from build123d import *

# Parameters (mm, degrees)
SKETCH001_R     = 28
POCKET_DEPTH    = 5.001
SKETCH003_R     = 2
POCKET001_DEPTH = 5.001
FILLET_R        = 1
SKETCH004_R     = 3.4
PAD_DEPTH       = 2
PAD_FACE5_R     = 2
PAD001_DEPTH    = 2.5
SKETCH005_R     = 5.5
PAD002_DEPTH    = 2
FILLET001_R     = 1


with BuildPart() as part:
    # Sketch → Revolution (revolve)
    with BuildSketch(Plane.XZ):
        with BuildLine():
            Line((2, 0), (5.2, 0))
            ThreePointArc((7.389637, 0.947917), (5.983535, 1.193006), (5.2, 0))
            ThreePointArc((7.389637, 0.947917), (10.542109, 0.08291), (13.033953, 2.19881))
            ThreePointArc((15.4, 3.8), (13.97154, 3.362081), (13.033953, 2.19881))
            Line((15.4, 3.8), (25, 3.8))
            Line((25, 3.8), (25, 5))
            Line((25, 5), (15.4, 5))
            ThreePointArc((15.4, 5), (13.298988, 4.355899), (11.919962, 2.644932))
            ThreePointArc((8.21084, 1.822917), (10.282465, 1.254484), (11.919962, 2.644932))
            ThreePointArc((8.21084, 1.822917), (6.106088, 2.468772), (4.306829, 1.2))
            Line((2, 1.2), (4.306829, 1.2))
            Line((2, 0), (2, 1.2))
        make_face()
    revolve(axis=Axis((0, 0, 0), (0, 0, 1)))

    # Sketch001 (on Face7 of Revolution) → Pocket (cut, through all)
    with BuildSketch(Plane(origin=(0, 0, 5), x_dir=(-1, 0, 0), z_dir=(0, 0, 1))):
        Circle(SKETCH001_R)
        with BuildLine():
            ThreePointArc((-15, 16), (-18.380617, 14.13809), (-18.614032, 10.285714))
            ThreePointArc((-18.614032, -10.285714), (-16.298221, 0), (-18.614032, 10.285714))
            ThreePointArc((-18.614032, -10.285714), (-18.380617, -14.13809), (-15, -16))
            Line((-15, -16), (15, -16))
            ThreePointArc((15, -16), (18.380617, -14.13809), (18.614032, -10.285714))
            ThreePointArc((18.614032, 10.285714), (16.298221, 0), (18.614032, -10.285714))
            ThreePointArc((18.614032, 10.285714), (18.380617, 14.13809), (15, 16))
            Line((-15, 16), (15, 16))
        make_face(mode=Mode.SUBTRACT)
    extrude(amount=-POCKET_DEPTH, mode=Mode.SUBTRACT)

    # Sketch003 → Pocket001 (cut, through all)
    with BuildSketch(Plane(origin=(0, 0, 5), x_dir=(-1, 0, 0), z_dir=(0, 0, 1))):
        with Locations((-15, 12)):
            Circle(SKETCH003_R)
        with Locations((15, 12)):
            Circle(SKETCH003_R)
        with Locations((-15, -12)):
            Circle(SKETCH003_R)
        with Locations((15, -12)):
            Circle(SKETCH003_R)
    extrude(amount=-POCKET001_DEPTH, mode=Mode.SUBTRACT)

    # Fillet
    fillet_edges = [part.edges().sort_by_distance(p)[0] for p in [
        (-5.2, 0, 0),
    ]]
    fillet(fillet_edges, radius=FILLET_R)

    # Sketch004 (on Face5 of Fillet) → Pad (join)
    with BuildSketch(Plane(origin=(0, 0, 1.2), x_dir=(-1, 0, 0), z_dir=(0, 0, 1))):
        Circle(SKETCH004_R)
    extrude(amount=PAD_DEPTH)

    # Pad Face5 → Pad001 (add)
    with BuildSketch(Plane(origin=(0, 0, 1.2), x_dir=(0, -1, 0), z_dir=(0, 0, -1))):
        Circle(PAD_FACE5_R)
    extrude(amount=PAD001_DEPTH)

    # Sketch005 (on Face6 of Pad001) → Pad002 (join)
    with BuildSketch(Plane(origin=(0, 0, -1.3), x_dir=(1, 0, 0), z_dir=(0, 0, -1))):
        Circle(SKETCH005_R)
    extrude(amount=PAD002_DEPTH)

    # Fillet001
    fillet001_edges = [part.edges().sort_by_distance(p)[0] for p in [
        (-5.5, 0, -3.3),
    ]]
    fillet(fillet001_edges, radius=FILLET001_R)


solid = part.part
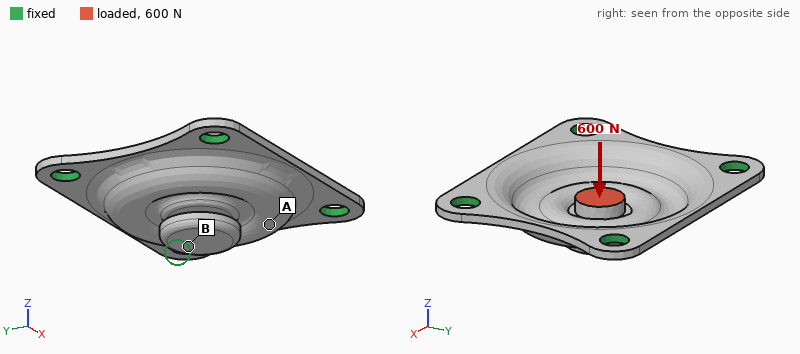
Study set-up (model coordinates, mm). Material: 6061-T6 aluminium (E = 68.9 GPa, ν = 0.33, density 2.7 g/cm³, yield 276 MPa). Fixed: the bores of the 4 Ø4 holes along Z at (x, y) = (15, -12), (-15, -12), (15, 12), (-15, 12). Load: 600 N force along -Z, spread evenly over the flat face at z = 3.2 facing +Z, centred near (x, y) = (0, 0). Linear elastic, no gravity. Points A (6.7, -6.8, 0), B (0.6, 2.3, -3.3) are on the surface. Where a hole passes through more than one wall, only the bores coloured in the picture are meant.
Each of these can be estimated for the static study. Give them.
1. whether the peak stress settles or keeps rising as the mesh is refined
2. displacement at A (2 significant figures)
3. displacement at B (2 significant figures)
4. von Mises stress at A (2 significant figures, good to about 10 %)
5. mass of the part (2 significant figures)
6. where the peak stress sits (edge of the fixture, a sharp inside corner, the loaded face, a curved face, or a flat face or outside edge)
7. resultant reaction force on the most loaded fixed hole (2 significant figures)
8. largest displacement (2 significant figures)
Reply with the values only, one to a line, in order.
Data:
keeps rising
36 µm
88 µm
94 MPa
4.7 g
edge of the fixture
330 N
89 µm
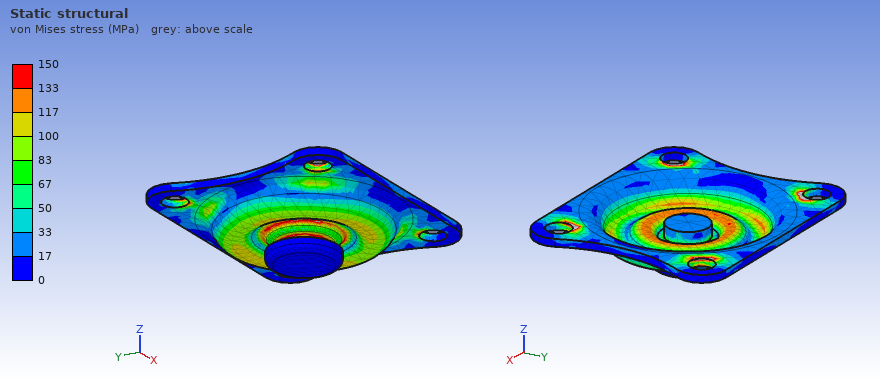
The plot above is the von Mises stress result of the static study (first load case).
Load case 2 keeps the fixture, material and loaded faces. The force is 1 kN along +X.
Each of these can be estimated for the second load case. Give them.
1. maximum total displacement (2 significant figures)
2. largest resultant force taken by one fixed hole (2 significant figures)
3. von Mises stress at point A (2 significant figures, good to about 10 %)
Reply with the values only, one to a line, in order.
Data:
59 µm
260 N
64 MPa
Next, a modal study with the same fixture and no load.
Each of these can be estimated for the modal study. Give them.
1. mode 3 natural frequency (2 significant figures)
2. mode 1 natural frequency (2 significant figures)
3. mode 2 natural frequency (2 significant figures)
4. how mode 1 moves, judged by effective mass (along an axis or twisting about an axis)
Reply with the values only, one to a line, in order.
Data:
17 kHz
11 kHz
15 kHz
along Z
